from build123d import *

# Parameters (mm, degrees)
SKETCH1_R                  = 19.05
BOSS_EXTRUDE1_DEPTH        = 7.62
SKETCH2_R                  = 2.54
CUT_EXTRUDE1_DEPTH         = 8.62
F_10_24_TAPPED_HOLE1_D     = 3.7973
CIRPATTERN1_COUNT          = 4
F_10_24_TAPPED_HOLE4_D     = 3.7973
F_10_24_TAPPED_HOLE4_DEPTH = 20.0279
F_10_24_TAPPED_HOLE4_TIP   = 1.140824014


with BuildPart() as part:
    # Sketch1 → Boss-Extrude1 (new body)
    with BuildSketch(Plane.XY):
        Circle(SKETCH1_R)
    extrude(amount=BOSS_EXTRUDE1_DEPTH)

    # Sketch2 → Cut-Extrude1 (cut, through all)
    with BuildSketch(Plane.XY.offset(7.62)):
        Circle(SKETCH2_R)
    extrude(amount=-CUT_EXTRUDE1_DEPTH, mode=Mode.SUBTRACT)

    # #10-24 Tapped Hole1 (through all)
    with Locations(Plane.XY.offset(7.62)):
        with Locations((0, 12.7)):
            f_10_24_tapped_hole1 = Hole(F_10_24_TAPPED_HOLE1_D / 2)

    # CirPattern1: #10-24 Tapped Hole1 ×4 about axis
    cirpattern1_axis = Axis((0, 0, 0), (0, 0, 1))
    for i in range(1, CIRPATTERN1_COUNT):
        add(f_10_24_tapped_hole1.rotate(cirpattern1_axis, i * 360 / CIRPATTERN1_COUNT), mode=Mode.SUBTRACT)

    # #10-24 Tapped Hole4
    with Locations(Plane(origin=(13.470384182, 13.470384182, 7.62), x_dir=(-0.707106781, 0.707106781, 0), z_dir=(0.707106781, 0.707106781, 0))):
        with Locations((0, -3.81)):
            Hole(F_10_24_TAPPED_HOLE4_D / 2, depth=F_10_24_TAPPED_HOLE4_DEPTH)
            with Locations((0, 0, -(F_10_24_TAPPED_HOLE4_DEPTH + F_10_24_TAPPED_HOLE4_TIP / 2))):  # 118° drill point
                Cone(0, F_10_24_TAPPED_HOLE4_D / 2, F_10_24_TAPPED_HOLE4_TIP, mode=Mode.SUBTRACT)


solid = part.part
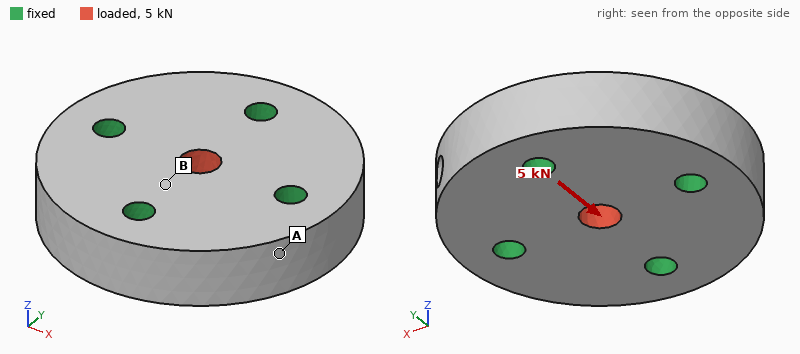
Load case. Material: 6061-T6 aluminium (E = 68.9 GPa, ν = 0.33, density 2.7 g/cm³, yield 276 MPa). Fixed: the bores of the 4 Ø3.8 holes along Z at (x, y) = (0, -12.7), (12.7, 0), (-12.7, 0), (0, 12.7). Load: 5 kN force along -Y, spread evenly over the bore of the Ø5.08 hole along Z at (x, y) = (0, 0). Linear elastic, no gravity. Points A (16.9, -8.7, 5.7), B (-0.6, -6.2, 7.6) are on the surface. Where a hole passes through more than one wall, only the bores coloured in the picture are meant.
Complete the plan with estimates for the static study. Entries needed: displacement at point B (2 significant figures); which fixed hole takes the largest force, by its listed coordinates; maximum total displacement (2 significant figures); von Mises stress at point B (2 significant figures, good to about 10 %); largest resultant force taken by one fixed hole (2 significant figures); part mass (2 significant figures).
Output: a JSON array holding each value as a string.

["2.7 µm", "(0, -12.7)", "5.1 µm", "40 MPa", "1.8 kN", "22 g"]
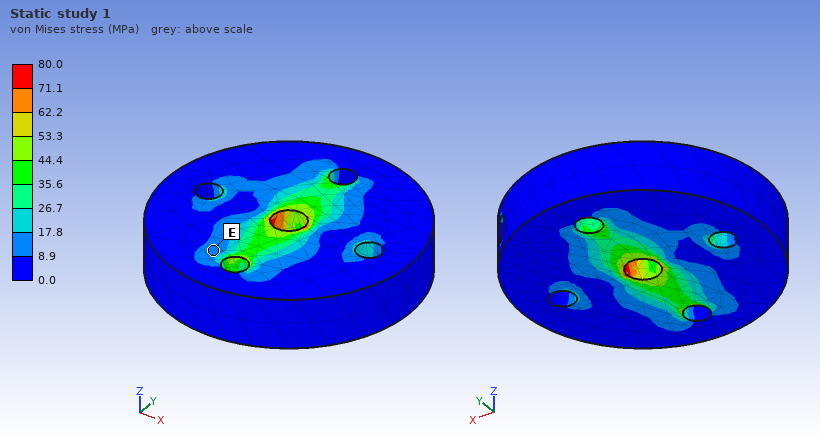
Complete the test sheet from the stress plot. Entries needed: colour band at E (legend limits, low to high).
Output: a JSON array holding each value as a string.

["8.9 to 17.8 MPa"]
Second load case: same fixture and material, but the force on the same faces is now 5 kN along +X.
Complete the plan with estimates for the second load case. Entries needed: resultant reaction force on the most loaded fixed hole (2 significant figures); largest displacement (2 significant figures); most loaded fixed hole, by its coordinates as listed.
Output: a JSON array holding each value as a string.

["1.8 kN", "5.1 µm", "(-12.7, 0)"]
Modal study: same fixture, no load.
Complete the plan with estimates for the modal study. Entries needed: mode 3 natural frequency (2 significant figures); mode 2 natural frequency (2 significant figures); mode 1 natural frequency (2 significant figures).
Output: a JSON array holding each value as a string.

["49 kHz", "48 kHz", "46 kHz"]
